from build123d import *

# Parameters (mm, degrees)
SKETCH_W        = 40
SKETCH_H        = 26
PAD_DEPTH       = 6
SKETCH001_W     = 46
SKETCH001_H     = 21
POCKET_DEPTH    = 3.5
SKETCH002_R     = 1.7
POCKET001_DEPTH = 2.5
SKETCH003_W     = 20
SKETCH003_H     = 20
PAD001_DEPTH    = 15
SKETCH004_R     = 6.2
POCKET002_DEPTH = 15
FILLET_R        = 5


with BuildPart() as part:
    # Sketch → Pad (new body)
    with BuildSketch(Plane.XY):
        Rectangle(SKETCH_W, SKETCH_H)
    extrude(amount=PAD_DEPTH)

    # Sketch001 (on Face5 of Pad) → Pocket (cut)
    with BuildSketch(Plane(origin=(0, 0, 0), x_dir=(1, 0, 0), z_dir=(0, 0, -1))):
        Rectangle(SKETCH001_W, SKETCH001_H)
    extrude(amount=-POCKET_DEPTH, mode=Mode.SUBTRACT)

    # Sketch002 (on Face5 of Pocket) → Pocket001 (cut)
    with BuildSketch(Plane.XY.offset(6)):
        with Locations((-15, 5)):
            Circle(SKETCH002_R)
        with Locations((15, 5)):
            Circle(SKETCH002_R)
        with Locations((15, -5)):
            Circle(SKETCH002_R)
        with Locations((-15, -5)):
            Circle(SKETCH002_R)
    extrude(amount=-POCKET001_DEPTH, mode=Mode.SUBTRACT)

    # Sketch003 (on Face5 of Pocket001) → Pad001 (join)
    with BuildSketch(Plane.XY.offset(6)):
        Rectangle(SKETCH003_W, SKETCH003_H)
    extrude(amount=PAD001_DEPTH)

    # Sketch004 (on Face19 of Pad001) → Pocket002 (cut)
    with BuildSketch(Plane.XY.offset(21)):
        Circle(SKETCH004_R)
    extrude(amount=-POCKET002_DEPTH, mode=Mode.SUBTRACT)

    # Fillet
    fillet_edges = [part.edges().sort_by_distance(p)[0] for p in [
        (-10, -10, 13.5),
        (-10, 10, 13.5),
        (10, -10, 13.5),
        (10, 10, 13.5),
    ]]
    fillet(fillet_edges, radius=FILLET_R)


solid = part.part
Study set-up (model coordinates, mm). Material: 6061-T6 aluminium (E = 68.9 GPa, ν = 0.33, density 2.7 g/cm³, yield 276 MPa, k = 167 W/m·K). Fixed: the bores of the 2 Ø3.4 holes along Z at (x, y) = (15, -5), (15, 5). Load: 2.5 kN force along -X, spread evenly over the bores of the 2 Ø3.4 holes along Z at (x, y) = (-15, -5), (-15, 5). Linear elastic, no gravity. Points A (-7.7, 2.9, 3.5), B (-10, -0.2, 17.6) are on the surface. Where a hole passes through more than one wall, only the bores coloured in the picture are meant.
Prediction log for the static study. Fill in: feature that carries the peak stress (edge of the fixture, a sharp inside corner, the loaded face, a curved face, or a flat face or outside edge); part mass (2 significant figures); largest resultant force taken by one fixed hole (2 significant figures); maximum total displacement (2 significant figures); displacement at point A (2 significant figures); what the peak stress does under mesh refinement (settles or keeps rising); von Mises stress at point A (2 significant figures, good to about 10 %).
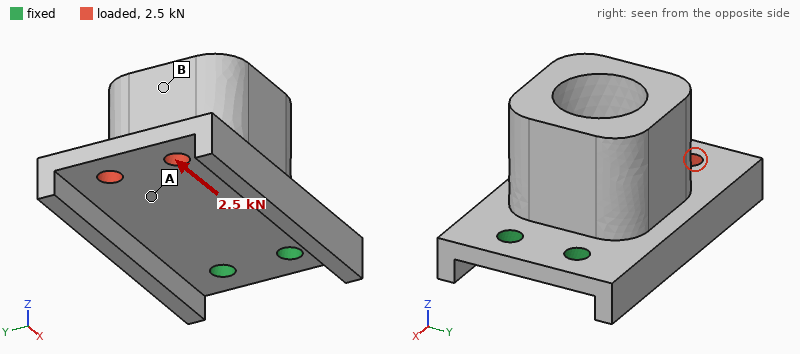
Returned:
edge of the fixture
19 g
1.3 kN
20 µm
13 µm
keeps rising
46 MPa
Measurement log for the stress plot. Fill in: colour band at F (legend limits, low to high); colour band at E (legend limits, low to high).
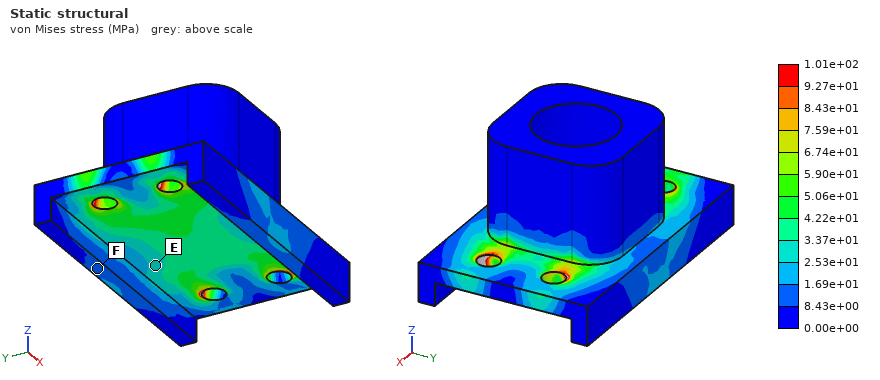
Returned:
8.43e+00 to 1.69e+01 MPa
2.53e+01 to 3.37e+01 MPa
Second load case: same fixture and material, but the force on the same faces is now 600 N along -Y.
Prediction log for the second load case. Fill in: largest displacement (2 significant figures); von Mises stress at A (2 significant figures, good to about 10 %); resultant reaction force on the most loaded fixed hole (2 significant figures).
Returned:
60 µm
19 MPa
1.4 kN
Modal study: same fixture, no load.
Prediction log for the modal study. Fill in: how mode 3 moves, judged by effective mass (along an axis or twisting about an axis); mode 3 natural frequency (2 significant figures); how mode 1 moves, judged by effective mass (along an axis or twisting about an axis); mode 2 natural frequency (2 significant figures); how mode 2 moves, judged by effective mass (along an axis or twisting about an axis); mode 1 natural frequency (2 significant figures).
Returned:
along Y
7600 Hz
along Z
5500 Hz
along Y
1700 Hz
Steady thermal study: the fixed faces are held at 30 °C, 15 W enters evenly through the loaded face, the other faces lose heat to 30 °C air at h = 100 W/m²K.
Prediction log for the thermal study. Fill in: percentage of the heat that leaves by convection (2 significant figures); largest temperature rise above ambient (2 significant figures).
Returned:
30 %
25 K
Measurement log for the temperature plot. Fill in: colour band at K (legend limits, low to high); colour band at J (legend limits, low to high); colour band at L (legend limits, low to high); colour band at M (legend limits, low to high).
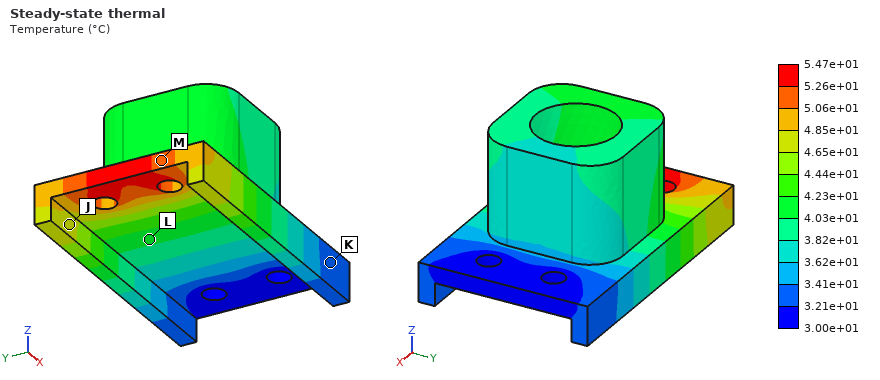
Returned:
3.21e+01 to 3.41e+01 °C
4.65e+01 to 4.85e+01 °C
4.03e+01 to 4.23e+01 °C
5.06e+01 to 5.26e+01 °C
